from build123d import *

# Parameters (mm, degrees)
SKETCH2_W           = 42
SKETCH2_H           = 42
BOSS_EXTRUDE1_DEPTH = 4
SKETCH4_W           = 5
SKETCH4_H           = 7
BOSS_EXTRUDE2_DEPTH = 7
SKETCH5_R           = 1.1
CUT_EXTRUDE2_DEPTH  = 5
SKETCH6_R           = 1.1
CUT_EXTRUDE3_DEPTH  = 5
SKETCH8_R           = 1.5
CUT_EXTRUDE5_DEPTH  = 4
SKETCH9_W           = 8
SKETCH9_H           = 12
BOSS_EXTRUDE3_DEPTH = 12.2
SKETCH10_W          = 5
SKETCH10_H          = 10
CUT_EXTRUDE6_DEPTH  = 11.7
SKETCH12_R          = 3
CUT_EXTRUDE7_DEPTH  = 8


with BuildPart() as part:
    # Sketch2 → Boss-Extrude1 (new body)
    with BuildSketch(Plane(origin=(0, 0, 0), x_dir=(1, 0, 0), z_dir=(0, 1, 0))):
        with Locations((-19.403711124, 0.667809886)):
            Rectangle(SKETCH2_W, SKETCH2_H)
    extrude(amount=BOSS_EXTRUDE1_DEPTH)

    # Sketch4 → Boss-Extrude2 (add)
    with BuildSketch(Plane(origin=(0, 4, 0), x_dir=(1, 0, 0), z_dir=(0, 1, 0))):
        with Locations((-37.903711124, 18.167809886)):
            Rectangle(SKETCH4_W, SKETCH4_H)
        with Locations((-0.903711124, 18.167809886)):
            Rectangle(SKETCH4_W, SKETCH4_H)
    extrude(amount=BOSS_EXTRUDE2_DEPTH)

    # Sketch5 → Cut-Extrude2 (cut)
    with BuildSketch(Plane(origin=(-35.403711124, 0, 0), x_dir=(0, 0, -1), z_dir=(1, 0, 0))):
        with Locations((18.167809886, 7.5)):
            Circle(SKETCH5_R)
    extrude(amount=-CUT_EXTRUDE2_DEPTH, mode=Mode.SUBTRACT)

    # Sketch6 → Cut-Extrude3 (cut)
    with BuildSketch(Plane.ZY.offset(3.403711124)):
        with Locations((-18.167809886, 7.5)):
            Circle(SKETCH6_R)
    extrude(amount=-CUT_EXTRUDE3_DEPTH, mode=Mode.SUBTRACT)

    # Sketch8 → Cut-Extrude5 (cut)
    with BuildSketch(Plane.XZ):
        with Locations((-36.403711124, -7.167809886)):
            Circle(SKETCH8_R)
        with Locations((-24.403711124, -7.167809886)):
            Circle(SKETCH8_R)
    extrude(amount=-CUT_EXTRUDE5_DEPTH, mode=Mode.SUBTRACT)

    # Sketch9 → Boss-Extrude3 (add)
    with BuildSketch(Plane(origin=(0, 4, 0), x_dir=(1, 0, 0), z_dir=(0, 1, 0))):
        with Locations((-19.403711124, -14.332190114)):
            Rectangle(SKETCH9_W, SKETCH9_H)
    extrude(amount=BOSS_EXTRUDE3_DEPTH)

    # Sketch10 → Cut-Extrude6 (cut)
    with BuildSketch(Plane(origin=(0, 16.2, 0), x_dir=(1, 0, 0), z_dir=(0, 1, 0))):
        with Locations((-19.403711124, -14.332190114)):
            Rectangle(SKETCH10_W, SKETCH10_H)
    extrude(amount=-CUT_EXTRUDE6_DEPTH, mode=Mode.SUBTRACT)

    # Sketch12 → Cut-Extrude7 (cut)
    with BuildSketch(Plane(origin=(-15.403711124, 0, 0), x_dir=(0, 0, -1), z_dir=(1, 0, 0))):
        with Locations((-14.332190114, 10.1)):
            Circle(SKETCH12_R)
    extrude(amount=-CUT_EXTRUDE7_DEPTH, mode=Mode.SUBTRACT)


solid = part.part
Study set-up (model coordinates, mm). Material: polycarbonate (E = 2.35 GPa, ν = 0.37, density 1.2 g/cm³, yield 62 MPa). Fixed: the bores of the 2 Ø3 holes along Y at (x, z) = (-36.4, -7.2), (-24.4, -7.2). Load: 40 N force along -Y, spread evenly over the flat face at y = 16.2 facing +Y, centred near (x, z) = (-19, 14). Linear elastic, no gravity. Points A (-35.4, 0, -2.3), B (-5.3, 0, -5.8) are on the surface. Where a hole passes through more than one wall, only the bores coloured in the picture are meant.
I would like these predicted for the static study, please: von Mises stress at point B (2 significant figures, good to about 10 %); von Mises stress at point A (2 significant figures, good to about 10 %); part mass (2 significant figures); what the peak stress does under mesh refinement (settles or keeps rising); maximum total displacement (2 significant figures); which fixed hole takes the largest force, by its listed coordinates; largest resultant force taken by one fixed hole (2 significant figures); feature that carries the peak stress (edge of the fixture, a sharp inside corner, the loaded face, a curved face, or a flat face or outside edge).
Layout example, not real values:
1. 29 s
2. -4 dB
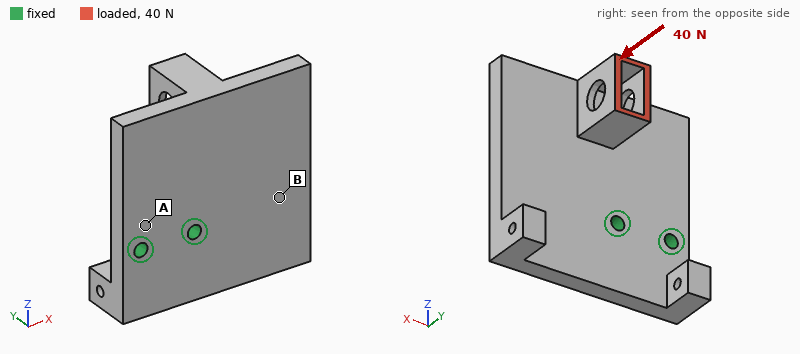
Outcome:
1. 2.8 MPa
2. 7.3 MPa
3. 9.5 g
4. keeps rising
5. 0.69 mm
6. (-24.4, -7.2)
7. 44 N
8. edge of the fixture
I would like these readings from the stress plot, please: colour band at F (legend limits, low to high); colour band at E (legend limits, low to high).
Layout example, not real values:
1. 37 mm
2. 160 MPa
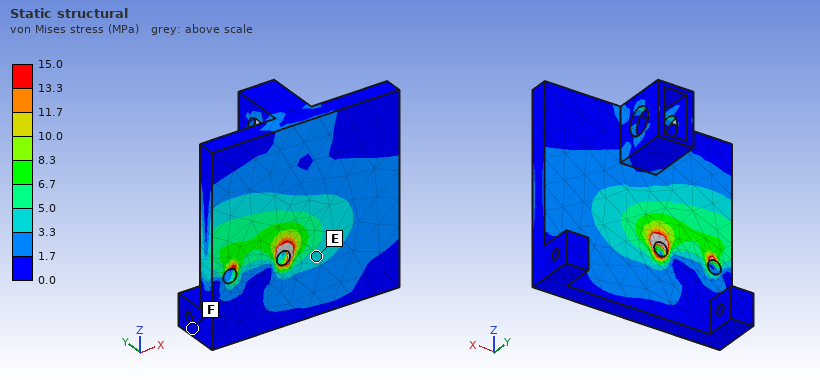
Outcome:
1. 0.0 to 1.7 MPa
2. 3.3 to 5.0 MPa
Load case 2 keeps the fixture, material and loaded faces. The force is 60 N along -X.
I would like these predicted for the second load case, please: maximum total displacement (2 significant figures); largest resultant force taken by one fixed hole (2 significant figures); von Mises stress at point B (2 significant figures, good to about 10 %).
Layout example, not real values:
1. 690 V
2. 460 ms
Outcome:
1. 0.71 mm
2. 110 N
3. 2.6 MPa
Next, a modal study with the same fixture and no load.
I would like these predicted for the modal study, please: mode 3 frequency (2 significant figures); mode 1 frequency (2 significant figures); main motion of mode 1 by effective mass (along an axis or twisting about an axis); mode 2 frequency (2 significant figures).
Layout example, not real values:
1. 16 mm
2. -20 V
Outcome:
1. 1800 Hz
2. 780 Hz
3. along Y
4. 1100 Hz
